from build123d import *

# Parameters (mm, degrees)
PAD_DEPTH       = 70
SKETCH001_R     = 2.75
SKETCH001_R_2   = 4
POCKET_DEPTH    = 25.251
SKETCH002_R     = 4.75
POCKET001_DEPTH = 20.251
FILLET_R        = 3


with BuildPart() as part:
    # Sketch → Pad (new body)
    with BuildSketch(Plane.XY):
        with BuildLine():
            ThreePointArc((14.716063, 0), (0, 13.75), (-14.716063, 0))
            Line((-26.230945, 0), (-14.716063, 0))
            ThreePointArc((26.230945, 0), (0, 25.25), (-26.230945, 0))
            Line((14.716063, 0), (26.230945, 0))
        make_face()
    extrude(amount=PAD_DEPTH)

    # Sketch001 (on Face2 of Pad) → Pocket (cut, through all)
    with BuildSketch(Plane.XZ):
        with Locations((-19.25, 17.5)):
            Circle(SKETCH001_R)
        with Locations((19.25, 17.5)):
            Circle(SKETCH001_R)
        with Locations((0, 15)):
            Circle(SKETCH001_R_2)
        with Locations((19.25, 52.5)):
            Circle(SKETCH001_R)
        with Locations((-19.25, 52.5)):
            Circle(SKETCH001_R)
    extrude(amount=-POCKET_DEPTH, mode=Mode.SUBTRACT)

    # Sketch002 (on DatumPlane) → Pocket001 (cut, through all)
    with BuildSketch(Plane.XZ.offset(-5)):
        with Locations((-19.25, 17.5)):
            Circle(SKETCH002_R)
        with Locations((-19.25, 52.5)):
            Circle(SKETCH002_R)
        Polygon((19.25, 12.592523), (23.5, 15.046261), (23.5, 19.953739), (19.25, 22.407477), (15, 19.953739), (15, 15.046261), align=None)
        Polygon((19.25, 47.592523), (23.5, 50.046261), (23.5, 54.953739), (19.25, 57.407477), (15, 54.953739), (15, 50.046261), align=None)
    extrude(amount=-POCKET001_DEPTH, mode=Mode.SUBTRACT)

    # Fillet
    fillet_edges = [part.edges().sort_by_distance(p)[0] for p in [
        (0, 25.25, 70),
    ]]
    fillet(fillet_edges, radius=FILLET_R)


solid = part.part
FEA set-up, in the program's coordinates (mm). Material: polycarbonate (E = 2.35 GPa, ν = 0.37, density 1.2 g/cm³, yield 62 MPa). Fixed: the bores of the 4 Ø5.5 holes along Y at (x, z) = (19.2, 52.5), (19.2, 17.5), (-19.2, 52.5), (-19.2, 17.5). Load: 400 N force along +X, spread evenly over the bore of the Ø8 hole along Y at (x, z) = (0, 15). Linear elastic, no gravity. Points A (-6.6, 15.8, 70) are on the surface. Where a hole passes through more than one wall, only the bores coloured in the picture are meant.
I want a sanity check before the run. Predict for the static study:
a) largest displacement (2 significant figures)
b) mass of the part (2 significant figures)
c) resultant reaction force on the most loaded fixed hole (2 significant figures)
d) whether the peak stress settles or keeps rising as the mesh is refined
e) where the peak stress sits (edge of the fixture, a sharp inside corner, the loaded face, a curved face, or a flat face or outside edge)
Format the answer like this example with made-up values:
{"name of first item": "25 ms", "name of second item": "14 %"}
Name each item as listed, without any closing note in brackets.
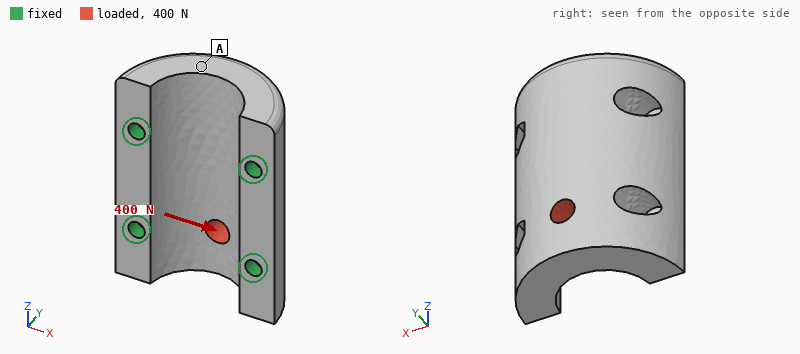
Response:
{"largest displacement": "39 µm", "mass of the part": "55 g", "resultant reaction force on the most loaded fixed hole": "180 N", "whether the peak stress settles or keeps rising as the mesh is refined": "keeps rising", "where the peak stress sits": "edge of the fixture"}
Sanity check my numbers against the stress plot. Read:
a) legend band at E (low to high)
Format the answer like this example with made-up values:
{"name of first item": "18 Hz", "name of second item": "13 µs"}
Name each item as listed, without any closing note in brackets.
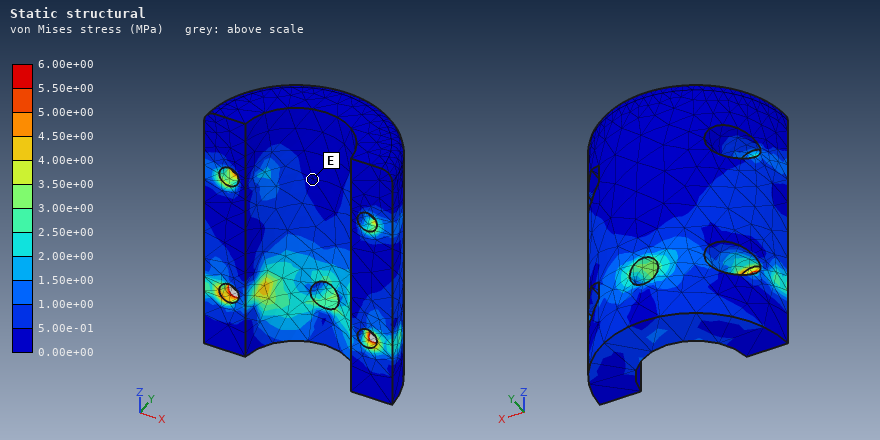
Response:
{"legend band at E": "0.00e+00 to 5.00e-01 MPa"}
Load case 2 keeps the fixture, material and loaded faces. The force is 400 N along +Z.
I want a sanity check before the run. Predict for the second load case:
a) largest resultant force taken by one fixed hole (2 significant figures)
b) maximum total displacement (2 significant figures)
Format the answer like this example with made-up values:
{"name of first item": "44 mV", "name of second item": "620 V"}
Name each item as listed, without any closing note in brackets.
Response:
{"largest resultant force taken by one fixed hole": "140 N", "maximum total displacement": "47 µm"}
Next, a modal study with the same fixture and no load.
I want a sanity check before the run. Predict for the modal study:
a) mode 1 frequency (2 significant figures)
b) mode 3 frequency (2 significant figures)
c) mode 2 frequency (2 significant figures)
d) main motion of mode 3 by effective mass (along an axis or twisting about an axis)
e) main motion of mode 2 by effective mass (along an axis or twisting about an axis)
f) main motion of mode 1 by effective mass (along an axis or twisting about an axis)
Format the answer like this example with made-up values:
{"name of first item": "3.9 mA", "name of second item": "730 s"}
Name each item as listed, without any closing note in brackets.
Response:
{"mode 1 frequency": "3200 Hz", "mode 3 frequency": "4200 Hz", "mode 2 frequency": "3700 Hz", "main motion of mode 3 by effective mass": "twisting about Y", "main motion of mode 2 by effective mass": "along X", "main motion of mode 1 by effective mass": "along Z"}
